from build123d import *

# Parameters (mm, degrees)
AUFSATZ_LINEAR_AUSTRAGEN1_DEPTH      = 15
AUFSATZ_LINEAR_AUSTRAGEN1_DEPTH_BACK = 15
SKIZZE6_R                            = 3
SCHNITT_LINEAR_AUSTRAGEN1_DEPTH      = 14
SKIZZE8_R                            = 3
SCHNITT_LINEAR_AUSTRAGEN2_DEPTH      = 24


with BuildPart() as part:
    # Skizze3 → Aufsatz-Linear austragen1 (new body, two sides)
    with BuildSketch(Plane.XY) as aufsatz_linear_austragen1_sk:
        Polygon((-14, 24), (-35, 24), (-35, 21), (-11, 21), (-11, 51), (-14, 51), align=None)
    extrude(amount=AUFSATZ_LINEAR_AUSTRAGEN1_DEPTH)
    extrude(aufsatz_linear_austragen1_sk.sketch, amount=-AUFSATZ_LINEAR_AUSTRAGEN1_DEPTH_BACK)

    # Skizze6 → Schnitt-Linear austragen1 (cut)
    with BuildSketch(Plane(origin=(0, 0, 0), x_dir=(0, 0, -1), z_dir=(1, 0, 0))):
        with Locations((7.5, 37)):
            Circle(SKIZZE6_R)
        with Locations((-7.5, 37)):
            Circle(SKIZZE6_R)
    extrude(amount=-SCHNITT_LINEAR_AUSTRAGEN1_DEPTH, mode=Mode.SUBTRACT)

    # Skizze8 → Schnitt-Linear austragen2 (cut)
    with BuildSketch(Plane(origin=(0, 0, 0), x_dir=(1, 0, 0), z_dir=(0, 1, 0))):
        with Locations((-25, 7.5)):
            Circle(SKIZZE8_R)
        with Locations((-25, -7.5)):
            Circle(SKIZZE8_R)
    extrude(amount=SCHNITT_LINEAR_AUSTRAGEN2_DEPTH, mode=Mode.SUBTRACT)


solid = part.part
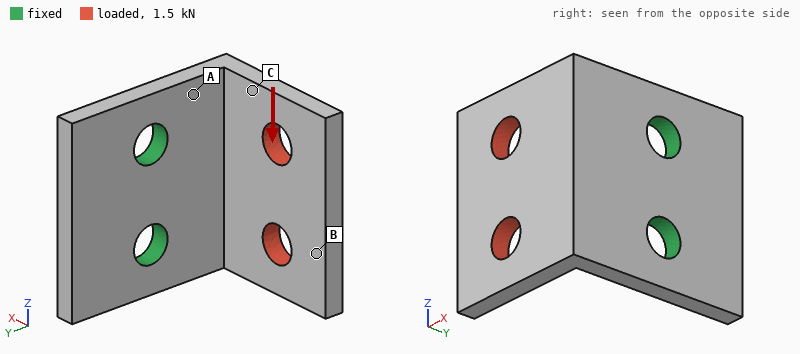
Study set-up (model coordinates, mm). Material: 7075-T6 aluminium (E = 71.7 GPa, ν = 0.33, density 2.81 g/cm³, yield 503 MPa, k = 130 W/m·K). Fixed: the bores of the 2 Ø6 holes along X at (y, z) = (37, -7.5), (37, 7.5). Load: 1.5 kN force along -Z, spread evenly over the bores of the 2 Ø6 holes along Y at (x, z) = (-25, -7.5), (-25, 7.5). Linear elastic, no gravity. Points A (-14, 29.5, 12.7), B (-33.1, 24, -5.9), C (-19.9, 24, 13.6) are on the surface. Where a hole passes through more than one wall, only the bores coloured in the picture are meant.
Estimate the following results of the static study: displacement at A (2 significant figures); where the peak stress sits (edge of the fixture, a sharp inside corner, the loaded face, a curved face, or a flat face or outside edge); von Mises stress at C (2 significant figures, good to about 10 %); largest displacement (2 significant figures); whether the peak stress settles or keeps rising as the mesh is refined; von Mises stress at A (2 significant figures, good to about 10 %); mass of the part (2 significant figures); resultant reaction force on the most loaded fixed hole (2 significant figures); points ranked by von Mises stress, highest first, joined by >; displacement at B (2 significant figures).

0.064 mm
edge of the fixture
92 MPa
0.38 mm
keeps rising
150 MPa
12 g
1.6 kN
A > C > B
0.30 mm
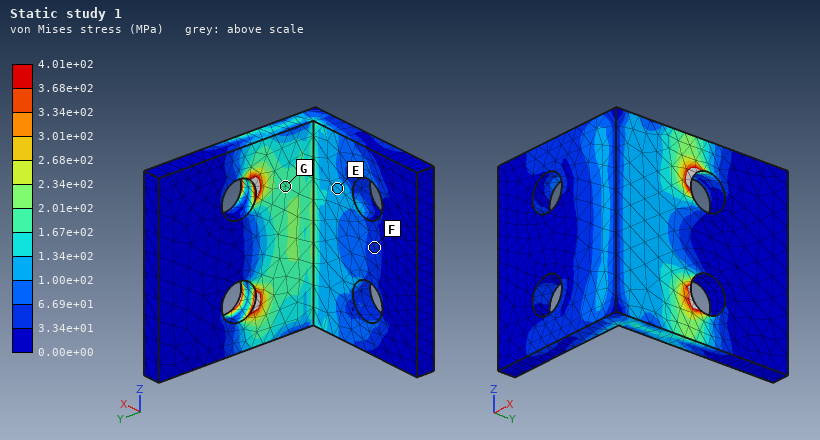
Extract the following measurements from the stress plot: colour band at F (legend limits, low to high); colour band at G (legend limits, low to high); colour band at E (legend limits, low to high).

3.34e+01 to 6.69e+01 MPa
1.67e+02 to 2.01e+02 MPa
1.00e+02 to 1.34e+02 MPa
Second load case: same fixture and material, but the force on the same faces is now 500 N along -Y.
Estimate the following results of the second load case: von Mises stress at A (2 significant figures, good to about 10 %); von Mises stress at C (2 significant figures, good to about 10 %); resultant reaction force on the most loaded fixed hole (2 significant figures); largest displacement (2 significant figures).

130 MPa
57 MPa
260 N
0.48 mm
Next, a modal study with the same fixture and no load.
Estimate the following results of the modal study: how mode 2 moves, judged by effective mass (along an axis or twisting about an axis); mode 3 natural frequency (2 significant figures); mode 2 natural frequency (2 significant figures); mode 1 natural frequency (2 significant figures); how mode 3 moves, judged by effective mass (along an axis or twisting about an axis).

along Z
8300 Hz
5000 Hz
2700 Hz
along X
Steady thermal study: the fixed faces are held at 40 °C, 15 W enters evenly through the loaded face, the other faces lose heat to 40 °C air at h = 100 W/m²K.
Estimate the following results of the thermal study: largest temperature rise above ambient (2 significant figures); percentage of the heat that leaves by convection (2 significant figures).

28 K
25 %
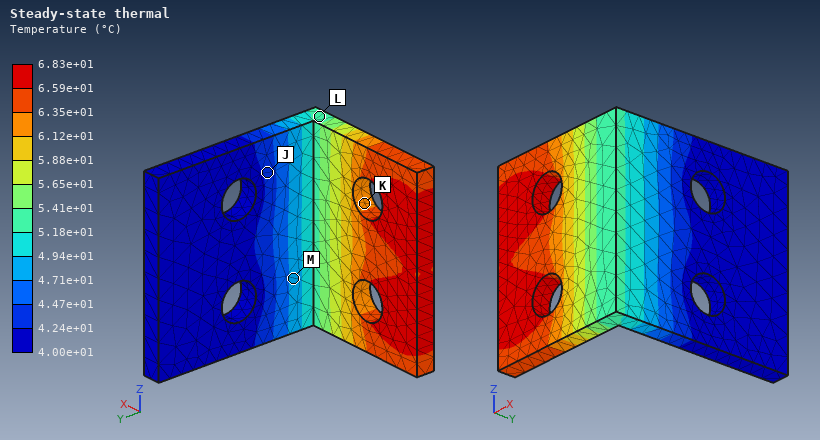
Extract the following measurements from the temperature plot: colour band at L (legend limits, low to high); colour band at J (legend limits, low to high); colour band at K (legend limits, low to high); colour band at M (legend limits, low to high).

5.18e+01 to 5.41e+01 °C
4.24e+01 to 4.47e+01 °C
6.12e+01 to 6.35e+01 °C
4.71e+01 to 4.94e+01 °C
